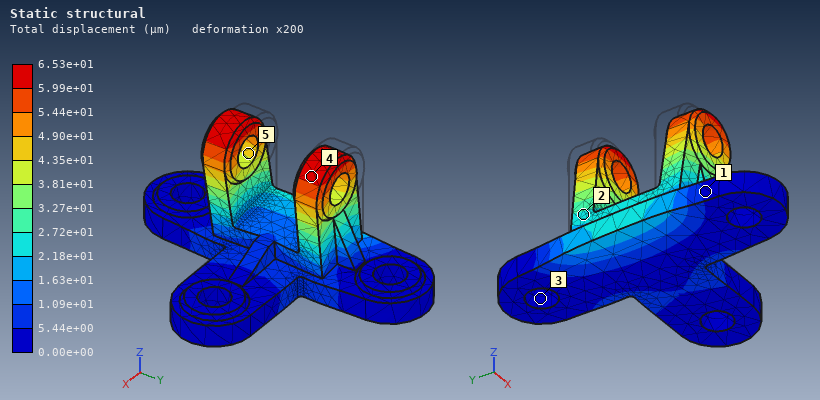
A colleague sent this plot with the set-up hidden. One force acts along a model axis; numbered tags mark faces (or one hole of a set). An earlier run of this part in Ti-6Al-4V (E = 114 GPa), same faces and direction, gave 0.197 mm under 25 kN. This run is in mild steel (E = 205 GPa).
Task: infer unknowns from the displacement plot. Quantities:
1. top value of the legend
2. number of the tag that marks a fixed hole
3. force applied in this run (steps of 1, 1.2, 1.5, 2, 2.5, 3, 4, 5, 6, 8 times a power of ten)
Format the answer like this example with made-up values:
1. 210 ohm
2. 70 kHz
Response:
1. 6.53e+01 µm
2. 3
3. 15 kN
